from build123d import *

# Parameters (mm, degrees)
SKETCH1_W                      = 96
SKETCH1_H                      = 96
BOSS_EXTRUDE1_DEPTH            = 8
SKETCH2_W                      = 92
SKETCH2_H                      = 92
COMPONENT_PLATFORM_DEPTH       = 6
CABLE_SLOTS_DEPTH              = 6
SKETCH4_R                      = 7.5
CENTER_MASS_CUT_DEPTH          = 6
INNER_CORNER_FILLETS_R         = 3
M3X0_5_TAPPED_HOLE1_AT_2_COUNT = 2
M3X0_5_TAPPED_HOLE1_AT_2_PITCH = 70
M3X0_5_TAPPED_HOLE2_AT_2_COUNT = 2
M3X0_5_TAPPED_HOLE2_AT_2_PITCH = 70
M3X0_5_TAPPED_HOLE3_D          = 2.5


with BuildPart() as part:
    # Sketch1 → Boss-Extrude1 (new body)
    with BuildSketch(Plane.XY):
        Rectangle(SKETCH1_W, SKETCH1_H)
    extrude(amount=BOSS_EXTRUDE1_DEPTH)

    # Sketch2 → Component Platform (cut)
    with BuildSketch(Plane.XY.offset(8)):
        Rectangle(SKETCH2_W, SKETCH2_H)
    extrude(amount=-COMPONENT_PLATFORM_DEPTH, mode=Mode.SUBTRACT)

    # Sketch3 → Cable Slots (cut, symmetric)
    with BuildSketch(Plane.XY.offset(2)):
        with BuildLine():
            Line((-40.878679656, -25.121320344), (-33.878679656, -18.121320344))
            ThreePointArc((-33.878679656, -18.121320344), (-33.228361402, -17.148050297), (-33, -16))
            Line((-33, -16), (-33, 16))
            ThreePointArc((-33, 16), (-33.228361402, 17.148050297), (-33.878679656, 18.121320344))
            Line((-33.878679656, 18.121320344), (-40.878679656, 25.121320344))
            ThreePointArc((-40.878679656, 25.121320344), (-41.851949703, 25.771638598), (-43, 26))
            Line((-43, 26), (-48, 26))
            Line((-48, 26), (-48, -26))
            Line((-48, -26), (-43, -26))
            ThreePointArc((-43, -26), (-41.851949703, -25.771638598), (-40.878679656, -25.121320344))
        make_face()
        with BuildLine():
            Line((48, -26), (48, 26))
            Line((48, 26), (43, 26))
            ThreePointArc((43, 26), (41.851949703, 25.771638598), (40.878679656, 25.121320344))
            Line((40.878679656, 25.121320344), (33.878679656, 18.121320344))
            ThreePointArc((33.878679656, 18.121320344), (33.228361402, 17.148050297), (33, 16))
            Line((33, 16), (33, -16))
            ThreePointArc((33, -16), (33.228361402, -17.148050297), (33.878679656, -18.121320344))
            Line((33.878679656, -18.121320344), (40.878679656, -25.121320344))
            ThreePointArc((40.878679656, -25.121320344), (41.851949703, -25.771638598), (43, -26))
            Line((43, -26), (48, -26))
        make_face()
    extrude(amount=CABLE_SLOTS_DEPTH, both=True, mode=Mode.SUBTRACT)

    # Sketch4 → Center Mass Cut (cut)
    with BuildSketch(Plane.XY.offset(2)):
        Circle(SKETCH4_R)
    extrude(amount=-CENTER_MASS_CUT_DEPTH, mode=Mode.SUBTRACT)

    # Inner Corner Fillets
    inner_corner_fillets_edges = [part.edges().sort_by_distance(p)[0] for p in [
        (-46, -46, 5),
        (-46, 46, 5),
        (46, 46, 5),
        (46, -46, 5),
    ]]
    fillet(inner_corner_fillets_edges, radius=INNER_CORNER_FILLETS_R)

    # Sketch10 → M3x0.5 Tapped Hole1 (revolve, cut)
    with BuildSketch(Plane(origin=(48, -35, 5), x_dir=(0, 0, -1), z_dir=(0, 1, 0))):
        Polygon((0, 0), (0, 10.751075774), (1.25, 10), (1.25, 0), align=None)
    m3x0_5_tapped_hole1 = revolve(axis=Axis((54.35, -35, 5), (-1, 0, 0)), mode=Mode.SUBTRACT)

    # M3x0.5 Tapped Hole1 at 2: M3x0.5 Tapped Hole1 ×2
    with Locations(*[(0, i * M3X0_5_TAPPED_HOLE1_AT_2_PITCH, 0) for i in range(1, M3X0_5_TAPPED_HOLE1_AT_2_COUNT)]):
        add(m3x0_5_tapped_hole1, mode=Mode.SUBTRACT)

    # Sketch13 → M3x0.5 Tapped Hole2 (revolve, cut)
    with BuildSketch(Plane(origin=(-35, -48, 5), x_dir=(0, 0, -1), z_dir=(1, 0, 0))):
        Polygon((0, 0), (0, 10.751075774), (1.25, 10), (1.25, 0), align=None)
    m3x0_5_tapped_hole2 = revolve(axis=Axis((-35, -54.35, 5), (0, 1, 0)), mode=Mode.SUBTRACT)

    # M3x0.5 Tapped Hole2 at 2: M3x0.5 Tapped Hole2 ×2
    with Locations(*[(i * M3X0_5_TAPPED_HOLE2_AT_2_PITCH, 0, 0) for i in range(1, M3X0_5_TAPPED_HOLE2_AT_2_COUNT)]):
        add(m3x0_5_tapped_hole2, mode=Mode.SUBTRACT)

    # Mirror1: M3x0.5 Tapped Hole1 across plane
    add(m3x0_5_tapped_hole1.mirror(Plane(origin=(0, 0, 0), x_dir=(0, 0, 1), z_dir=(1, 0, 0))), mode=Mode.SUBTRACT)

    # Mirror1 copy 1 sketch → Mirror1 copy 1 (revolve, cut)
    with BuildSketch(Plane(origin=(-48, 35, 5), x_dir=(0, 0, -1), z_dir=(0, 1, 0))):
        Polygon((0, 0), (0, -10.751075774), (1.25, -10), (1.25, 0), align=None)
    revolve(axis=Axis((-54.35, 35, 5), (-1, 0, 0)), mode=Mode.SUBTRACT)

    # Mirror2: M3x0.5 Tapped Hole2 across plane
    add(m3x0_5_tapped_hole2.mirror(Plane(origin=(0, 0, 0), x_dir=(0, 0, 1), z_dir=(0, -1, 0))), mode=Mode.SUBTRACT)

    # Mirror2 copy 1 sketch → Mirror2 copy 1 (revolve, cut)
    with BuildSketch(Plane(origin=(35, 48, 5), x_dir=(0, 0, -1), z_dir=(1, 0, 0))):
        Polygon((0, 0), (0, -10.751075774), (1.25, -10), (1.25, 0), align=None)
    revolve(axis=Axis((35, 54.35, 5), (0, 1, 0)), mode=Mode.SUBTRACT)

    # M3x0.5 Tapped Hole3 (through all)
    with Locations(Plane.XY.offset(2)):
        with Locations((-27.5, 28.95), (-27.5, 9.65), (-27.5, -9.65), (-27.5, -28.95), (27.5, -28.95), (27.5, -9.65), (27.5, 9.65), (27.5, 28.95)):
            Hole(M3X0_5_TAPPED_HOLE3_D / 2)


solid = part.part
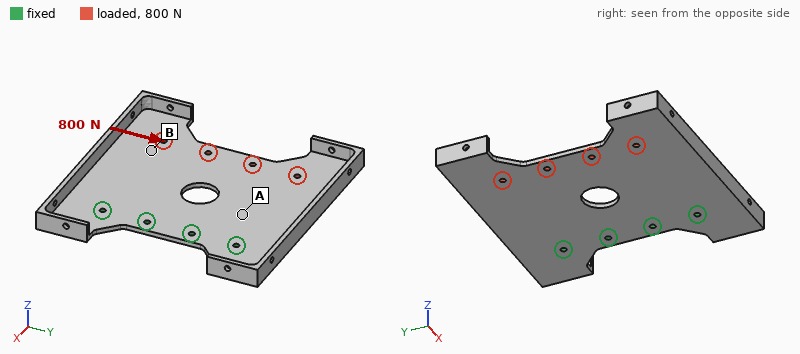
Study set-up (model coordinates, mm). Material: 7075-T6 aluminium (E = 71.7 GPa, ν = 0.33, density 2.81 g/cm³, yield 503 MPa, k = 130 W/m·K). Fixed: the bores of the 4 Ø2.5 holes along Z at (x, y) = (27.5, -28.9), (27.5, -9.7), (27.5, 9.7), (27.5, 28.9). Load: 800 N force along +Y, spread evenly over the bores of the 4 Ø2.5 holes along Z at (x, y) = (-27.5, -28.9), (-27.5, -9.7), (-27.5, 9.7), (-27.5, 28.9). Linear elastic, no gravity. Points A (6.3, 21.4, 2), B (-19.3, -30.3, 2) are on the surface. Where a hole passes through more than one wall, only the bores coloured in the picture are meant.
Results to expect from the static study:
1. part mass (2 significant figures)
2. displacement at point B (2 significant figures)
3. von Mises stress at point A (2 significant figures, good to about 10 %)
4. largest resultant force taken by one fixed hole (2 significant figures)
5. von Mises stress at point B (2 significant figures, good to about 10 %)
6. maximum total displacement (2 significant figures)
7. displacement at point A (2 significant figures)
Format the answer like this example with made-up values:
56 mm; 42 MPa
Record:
52 g; 23 µm; 15 MPa; 760 N; 5.6 MPa; 38 µm; 9.5 µm
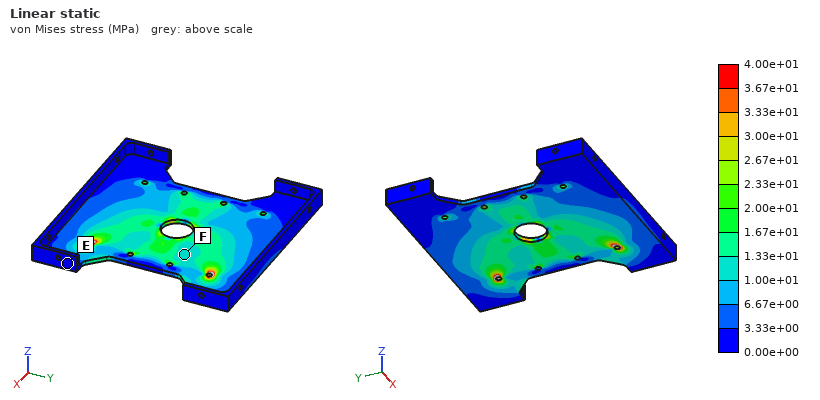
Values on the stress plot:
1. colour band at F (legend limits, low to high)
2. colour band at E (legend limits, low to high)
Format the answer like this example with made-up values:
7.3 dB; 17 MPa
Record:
1.00e+01 to 1.33e+01 MPa; 0.00e+00 to 3.33e+00 MPa
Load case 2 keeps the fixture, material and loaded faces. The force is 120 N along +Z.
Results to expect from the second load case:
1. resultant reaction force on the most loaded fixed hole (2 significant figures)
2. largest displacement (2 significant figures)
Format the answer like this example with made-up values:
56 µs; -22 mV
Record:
63 N; 1.4 mm
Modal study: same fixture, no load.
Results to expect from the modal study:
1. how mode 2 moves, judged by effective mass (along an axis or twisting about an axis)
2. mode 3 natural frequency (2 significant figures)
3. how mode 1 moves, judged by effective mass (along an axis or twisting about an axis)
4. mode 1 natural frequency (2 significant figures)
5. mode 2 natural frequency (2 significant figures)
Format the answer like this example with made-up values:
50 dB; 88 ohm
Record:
twisting about X; 1300 Hz; along Z; 370 Hz; 490 Hz
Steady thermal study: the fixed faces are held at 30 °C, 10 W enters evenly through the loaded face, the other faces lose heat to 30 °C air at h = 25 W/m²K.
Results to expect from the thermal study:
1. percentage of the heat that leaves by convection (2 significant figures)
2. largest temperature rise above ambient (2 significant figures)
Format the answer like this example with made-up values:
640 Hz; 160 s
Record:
40 %; 21 K
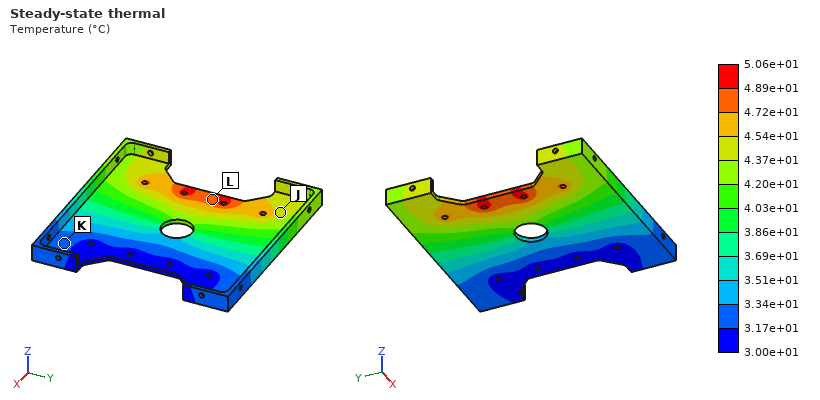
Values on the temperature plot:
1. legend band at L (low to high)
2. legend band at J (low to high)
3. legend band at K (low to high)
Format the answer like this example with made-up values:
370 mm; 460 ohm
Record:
4.72e+01 to 4.89e+01 °C; 4.37e+01 to 4.54e+01 °C; 3.17e+01 to 3.34e+01 °C
